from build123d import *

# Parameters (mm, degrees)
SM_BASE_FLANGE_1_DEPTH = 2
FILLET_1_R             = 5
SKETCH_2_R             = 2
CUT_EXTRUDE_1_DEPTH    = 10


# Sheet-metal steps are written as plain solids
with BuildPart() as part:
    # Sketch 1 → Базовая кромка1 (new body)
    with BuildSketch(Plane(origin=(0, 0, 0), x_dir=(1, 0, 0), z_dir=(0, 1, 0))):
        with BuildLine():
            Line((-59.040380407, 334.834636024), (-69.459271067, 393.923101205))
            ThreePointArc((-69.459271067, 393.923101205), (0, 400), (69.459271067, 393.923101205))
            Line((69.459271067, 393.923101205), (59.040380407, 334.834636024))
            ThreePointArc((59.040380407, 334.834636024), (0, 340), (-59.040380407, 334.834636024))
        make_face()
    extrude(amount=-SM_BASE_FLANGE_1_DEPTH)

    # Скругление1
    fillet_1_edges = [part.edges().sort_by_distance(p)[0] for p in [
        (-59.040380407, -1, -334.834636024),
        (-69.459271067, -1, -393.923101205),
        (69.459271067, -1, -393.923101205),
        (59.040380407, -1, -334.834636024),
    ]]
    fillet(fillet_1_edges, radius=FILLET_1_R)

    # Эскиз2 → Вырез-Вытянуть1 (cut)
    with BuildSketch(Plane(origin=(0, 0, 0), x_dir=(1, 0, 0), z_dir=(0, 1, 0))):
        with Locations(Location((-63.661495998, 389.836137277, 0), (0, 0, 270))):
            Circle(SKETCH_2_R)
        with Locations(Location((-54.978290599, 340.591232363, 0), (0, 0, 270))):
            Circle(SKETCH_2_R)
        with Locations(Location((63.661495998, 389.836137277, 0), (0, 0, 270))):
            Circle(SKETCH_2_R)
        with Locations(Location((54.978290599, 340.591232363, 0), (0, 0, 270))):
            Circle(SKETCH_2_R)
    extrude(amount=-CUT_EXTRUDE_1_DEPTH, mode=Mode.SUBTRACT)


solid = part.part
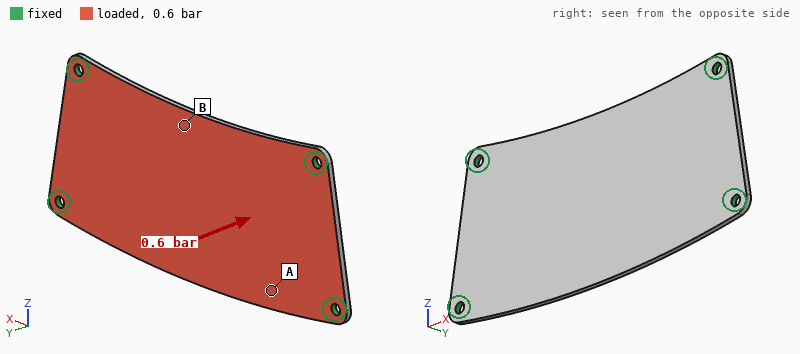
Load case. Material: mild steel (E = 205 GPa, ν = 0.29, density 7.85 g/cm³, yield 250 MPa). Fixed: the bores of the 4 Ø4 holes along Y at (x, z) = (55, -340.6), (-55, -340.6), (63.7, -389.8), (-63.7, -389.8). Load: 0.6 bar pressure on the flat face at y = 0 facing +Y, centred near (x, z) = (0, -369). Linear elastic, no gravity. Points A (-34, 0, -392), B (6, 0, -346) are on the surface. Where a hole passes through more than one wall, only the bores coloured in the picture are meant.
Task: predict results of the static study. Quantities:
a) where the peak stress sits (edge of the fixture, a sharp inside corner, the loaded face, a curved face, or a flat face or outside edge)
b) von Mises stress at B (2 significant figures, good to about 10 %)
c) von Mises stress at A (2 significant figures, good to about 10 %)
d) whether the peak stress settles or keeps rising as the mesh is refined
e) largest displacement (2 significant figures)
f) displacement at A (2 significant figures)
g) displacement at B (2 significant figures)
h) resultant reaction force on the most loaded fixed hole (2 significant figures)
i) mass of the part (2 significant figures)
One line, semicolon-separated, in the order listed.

edge of the fixture; 56 MPa; 29 MPa; keeps rising; 0.36 mm; 0.18 mm; 0.23 mm; 120 N; 120 g
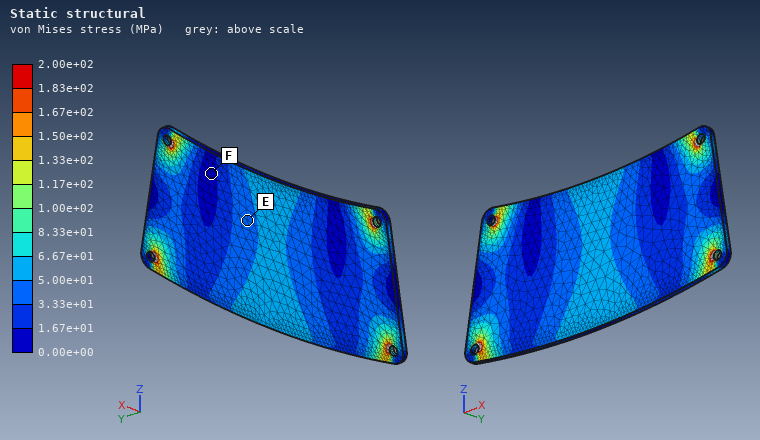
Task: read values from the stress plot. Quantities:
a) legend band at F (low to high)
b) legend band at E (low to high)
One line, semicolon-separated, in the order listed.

0.00e+00 to 1.67e+01 MPa; 3.33e+01 to 5.00e+01 MPa
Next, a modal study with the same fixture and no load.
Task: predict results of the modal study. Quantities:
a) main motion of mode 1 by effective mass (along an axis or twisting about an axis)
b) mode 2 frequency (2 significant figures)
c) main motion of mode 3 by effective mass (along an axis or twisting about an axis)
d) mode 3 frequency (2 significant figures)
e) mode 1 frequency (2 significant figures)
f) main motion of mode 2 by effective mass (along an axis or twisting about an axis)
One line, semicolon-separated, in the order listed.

along Y; 1300 Hz; twisting about Z; 1800 Hz; 660 Hz; twisting about X
